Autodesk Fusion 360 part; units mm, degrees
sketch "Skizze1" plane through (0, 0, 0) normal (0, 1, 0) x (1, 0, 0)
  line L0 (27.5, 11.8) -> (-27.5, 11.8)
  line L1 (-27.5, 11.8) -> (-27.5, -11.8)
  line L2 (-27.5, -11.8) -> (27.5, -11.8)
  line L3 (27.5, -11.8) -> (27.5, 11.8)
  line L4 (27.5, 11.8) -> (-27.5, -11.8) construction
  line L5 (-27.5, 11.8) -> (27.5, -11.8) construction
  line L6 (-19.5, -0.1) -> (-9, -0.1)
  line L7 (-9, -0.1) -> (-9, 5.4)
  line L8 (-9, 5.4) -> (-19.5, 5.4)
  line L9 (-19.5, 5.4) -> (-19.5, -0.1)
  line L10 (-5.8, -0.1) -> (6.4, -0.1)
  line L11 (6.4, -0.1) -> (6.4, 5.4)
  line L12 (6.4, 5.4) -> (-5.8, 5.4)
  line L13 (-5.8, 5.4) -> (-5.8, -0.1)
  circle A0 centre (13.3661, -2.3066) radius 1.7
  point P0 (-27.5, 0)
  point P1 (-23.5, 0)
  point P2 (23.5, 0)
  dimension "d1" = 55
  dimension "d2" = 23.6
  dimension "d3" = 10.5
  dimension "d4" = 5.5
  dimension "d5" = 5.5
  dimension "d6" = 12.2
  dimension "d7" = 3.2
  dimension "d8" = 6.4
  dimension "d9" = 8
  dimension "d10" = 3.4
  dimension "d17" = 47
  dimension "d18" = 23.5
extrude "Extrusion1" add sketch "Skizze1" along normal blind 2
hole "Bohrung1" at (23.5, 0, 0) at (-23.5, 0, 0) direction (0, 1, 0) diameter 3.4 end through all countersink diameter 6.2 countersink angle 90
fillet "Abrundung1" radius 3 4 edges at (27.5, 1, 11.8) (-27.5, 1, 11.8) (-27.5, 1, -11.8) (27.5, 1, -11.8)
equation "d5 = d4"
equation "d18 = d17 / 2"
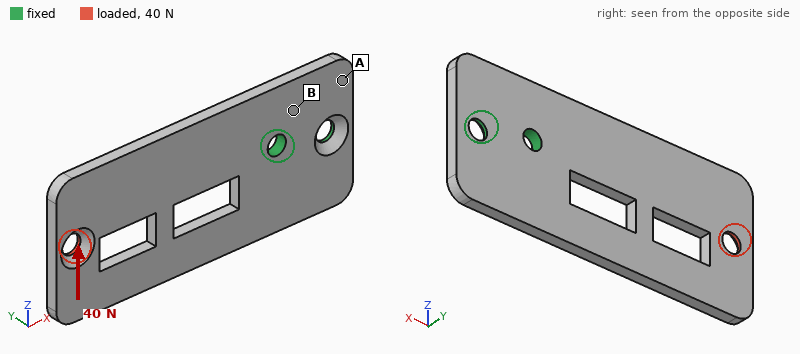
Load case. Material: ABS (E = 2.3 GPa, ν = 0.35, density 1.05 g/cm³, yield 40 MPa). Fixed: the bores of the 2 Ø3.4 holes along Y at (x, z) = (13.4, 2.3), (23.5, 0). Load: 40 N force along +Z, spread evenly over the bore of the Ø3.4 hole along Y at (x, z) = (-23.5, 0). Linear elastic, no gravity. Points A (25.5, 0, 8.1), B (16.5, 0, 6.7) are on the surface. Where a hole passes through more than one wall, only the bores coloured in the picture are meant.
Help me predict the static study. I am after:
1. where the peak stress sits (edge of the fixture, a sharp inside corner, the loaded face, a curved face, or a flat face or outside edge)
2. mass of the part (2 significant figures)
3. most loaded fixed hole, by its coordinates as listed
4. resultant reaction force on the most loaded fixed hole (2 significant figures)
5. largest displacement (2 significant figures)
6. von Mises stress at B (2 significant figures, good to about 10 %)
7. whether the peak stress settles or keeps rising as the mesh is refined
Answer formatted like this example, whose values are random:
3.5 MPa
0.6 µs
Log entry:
edge of the fixture
2.4 g
(13.4, 2.3)
140 N
0.65 mm
6.4 MPa
keeps rising
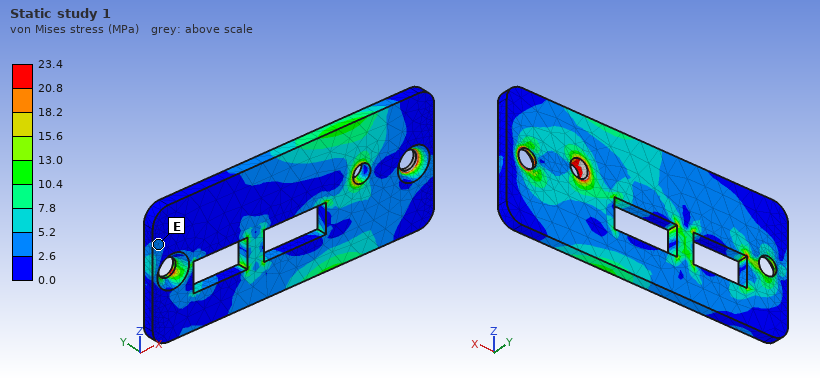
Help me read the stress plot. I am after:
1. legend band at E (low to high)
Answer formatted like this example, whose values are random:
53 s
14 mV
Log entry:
2.6 to 5.2 MPa
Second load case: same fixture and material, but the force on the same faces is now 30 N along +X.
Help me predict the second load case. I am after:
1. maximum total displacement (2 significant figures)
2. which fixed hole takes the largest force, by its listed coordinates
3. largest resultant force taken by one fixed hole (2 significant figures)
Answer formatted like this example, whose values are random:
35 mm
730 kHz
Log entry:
0.60 mm
(13.4, 2.3)
23 N
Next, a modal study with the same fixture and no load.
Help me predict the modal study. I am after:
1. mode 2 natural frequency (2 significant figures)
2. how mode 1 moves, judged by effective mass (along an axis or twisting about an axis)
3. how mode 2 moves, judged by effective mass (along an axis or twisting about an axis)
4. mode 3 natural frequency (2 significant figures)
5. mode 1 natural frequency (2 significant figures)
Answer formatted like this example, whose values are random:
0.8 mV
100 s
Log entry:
850 Hz
along Y
twisting about X
1700 Hz
280 Hz
